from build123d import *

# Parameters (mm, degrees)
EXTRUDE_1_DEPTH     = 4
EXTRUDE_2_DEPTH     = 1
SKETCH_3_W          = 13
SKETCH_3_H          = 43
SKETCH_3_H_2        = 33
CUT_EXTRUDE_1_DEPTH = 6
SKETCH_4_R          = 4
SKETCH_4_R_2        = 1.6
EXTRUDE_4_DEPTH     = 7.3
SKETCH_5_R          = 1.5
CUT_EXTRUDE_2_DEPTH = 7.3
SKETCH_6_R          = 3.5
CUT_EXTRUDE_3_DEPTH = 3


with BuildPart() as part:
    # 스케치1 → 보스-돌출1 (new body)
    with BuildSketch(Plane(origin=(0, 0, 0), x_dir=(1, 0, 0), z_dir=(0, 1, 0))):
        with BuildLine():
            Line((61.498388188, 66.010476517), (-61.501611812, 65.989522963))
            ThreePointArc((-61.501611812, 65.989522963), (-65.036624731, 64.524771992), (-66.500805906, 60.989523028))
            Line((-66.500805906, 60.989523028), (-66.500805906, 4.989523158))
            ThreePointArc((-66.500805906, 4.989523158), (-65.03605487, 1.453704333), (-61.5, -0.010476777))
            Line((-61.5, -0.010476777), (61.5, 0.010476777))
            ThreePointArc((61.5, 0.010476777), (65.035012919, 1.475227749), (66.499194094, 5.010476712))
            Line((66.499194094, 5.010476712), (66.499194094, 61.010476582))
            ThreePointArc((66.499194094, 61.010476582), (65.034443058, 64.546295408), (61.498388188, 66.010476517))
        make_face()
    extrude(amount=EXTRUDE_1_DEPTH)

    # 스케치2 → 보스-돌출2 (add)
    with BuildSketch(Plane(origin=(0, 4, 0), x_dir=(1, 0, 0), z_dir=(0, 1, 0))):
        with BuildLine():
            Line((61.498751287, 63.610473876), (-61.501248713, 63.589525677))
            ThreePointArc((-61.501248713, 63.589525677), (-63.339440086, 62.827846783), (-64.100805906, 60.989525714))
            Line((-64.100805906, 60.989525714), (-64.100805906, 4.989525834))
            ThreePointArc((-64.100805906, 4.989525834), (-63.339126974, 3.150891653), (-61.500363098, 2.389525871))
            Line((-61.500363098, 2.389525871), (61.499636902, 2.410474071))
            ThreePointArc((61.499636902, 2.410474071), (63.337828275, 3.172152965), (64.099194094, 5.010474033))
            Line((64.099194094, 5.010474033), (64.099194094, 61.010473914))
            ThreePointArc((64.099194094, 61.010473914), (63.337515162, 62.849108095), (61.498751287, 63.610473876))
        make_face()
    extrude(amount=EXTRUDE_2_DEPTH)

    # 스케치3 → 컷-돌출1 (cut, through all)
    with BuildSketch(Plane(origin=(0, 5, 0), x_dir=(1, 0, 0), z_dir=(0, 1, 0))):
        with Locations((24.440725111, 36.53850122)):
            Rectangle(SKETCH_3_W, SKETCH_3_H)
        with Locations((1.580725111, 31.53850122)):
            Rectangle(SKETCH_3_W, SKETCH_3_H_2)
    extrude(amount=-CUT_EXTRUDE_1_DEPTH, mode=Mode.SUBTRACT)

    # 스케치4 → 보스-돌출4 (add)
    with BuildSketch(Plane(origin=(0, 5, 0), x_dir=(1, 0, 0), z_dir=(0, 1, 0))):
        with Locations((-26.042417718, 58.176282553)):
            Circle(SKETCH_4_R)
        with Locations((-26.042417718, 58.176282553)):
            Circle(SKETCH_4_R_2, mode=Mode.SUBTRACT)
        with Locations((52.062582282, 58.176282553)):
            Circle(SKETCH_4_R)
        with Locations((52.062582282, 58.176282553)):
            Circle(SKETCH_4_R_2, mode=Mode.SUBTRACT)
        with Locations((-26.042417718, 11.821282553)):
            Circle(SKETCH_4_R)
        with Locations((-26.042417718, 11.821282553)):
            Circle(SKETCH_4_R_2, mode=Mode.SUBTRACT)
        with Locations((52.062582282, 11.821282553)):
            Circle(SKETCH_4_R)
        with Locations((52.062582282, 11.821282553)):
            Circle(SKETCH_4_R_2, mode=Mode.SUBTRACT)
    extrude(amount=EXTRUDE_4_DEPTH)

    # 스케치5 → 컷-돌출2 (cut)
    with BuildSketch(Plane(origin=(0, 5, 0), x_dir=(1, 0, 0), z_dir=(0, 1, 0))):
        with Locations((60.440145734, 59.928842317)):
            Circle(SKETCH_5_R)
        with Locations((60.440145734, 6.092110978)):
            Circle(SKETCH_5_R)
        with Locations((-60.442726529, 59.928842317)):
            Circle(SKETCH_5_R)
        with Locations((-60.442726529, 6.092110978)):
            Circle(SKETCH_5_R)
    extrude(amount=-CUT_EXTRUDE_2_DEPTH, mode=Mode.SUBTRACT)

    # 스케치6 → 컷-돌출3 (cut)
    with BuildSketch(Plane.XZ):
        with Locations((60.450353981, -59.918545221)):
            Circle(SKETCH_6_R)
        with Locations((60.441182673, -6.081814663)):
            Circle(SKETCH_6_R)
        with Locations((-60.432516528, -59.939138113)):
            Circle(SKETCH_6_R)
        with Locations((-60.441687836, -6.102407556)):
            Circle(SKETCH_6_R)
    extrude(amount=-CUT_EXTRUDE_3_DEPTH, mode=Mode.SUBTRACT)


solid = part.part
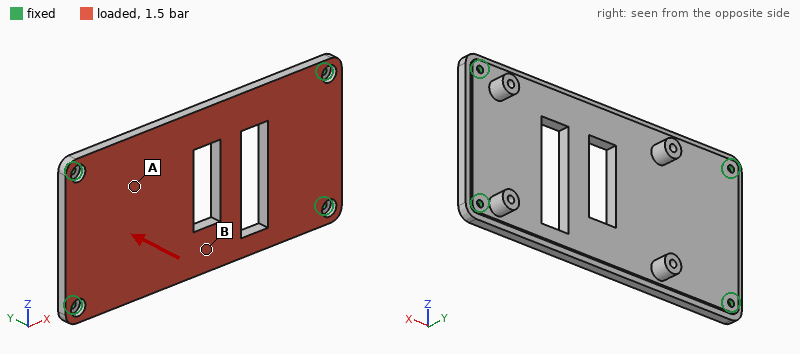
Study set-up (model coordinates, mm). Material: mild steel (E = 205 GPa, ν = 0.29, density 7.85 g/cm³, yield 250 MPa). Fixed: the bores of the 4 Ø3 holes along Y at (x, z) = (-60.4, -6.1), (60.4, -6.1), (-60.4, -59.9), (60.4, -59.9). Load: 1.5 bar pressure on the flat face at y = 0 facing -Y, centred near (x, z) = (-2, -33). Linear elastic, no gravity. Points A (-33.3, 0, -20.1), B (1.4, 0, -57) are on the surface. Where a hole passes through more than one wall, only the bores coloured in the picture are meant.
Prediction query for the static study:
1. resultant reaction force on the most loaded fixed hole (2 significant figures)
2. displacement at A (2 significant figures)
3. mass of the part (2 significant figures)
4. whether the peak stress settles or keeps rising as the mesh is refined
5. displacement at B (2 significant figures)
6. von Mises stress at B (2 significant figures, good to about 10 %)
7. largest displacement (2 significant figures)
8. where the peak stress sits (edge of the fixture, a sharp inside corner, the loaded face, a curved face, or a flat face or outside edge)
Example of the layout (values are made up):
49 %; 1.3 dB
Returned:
780 N; 0.059 mm; 300 g; keeps rising; 0.10 mm; 47 MPa; 0.11 mm; edge of the fixture
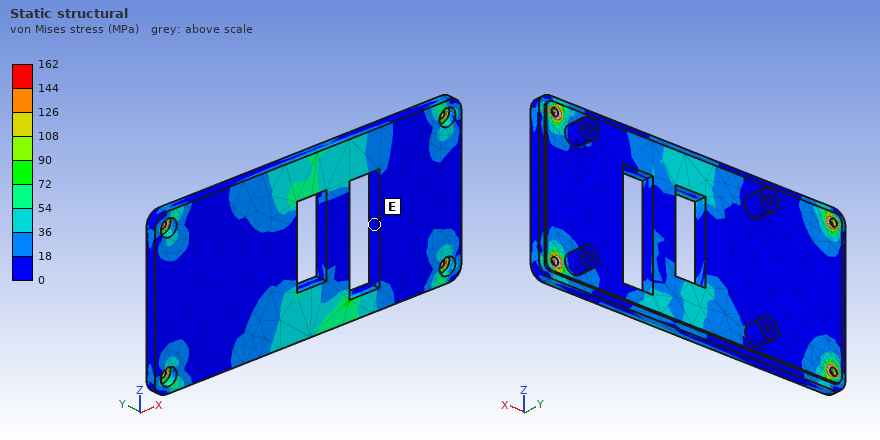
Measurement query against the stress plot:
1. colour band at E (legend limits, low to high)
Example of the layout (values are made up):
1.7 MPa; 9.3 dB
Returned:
0 to 18 MPa
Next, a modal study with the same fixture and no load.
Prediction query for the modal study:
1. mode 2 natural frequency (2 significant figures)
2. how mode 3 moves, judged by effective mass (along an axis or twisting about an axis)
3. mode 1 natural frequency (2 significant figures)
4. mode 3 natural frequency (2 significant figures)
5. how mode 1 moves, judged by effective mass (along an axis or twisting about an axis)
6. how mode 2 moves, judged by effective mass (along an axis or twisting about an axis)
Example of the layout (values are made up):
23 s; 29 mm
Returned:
2400 Hz; twisting about Z; 1100 Hz; 3000 Hz; along Y; twisting about X
